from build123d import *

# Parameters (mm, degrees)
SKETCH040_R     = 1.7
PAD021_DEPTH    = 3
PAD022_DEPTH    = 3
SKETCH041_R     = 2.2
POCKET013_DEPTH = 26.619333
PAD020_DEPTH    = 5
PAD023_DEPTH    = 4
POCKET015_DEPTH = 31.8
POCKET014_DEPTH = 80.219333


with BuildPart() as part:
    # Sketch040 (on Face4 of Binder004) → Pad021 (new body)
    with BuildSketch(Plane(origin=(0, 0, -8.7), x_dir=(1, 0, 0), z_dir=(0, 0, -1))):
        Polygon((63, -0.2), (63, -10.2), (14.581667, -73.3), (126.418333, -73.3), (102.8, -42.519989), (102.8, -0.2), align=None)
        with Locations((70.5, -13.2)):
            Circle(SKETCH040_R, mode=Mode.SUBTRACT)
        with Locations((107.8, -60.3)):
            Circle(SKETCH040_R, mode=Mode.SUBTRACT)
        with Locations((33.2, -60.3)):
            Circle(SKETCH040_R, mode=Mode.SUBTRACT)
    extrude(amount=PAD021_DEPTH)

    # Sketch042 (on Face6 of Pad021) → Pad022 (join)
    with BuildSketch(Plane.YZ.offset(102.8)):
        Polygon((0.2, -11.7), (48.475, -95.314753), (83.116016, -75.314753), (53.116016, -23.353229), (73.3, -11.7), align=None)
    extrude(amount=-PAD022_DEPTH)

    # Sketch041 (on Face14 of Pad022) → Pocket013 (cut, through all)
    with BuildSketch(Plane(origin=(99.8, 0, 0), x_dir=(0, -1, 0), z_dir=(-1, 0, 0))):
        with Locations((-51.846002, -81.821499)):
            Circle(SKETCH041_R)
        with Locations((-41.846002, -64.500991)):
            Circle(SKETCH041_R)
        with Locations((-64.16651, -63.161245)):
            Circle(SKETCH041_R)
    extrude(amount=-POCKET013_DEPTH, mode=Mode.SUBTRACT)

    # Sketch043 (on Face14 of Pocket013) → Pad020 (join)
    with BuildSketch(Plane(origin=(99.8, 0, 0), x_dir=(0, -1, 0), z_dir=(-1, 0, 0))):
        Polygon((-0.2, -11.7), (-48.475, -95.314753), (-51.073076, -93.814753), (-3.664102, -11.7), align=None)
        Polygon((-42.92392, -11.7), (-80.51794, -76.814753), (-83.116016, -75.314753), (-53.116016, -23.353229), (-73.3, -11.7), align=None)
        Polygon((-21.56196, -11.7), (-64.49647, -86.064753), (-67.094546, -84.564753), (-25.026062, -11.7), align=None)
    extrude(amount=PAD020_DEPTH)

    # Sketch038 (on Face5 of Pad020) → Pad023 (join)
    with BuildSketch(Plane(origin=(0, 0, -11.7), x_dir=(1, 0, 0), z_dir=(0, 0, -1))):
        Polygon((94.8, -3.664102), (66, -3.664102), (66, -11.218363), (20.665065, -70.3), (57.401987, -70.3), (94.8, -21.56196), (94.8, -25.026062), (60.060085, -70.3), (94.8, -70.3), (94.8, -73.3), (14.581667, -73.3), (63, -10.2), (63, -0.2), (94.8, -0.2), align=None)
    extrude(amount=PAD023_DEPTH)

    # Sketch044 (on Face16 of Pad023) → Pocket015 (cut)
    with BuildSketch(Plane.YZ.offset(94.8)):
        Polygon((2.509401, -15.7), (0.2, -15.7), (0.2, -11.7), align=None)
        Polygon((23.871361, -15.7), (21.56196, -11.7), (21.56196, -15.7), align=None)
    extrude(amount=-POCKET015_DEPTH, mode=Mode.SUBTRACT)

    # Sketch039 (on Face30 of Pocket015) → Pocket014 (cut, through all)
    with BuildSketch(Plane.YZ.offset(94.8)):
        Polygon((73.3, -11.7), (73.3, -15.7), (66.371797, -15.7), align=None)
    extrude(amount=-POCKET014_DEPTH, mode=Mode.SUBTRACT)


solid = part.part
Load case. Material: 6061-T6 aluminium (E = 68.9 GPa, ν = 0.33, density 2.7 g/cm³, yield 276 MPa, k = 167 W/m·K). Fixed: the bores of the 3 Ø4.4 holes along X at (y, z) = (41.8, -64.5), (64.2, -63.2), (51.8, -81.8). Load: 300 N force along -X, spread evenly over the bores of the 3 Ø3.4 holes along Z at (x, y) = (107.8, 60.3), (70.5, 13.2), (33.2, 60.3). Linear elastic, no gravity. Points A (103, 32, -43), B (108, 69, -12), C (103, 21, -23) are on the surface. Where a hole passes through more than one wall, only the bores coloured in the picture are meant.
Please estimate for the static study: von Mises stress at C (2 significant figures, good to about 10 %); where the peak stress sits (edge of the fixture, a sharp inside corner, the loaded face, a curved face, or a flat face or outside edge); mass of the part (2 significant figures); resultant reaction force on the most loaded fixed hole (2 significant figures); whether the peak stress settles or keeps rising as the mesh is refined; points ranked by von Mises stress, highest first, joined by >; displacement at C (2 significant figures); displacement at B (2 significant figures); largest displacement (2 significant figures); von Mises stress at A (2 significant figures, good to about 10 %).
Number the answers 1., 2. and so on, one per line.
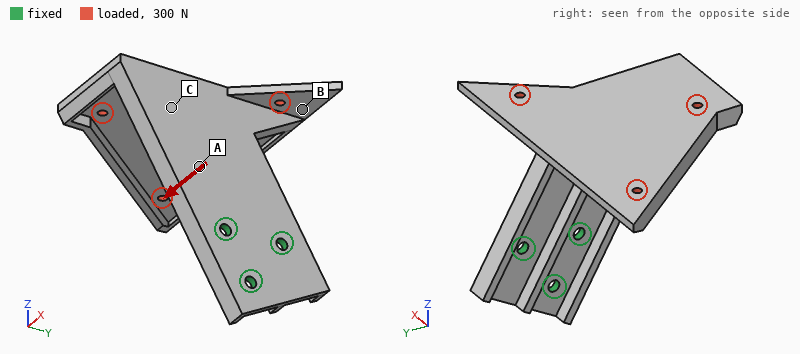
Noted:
1. 25 MPa
2. edge of the fixture
3. 85 g
4. 440 N
5. keeps rising
6. A > C > B
7. 0.33 mm
8. 0.85 mm
9. 1.9 mm
10. 43 MPa
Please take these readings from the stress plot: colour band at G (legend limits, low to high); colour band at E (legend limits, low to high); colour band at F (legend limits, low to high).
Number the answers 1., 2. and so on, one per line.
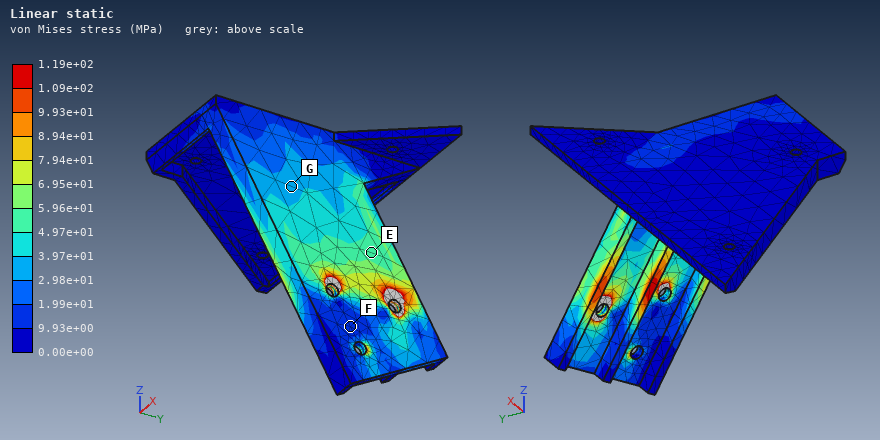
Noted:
1. 2.98e+01 to 3.97e+01 MPa
2. 4.97e+01 to 5.96e+01 MPa
3. 9.93e+00 to 1.99e+01 MPa
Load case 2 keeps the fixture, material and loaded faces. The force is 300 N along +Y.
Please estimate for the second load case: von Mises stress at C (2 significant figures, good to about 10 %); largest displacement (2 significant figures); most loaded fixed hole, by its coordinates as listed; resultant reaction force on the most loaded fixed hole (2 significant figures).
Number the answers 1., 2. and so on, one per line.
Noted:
1. 29 MPa
2. 1.5 mm
3. (41.8, -64.5)
4. 860 N
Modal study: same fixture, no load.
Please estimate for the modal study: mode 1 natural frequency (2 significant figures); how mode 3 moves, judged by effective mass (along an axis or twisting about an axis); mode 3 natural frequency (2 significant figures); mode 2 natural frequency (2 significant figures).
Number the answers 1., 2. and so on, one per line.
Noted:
1. 300 Hz
2. along X
3. 820 Hz
4. 490 Hz
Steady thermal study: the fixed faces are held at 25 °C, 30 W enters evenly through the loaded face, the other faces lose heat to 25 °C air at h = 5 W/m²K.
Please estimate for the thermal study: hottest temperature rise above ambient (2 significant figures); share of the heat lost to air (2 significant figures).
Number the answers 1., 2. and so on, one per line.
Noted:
1. 83 K
2. 16 %
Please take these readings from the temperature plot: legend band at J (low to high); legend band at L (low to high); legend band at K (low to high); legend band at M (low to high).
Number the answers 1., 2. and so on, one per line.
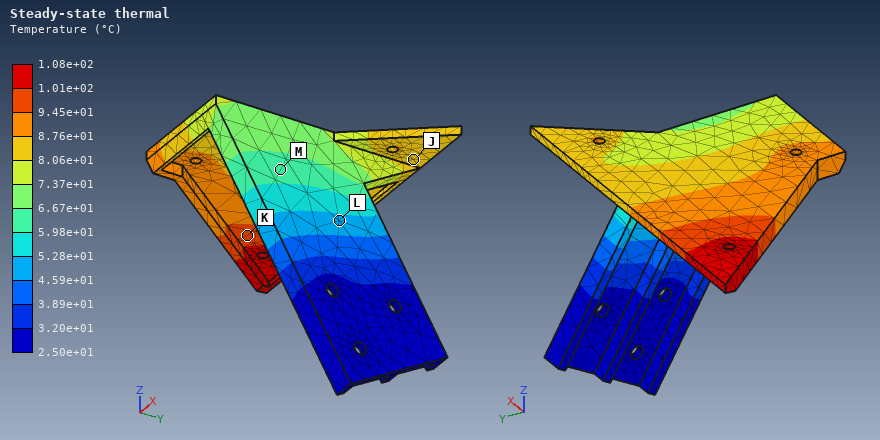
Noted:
1. 8.06e+01 to 8.76e+01 °C
2. 4.59e+01 to 5.28e+01 °C
3. 9.45e+01 to 1.01e+02 °C
4. 5.98e+01 to 6.67e+01 °C
